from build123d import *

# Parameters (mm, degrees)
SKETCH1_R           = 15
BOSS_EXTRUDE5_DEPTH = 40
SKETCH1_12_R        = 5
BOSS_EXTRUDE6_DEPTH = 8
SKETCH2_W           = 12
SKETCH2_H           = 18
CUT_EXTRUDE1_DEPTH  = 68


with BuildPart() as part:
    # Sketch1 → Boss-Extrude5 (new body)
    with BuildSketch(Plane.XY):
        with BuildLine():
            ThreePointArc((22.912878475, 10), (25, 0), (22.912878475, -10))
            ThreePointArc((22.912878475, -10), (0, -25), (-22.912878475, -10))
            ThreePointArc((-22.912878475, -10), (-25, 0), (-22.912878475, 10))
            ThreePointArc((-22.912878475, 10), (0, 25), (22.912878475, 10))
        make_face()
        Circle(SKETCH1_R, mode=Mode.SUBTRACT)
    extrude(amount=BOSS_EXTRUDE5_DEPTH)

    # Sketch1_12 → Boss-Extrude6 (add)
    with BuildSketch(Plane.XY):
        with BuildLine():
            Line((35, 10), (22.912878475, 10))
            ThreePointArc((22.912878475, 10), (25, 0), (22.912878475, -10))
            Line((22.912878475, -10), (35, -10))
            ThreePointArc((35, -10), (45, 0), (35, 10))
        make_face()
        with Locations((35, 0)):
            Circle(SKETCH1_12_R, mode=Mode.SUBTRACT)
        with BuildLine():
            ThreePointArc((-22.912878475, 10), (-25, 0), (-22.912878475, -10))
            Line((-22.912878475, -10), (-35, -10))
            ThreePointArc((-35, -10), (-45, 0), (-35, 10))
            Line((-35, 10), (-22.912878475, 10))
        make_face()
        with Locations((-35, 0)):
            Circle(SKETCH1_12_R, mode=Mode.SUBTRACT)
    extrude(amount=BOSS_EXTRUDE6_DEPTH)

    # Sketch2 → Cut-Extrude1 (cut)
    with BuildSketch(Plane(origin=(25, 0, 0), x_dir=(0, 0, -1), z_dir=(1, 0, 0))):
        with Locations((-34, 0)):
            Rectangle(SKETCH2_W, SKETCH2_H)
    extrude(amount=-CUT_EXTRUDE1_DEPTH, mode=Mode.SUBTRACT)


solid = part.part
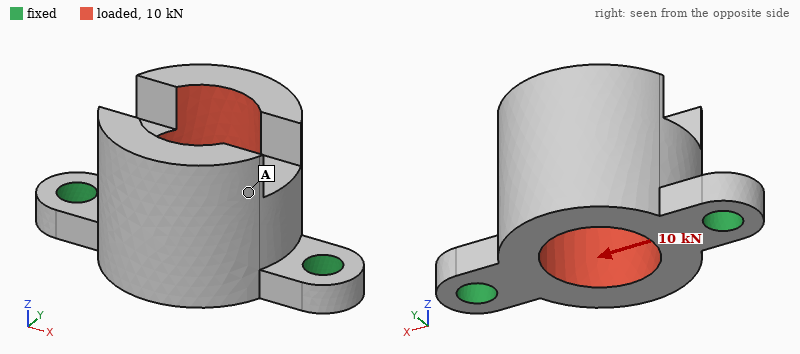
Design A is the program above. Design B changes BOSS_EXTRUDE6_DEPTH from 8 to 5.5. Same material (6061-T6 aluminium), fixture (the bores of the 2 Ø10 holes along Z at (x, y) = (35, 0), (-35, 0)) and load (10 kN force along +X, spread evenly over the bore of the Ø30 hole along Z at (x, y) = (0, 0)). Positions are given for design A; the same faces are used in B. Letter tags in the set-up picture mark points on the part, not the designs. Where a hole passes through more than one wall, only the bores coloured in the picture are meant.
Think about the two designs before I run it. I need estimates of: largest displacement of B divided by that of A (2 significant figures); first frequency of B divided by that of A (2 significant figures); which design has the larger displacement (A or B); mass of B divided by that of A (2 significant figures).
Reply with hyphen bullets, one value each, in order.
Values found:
- 1.5
- 0.68
- B
- 0.97
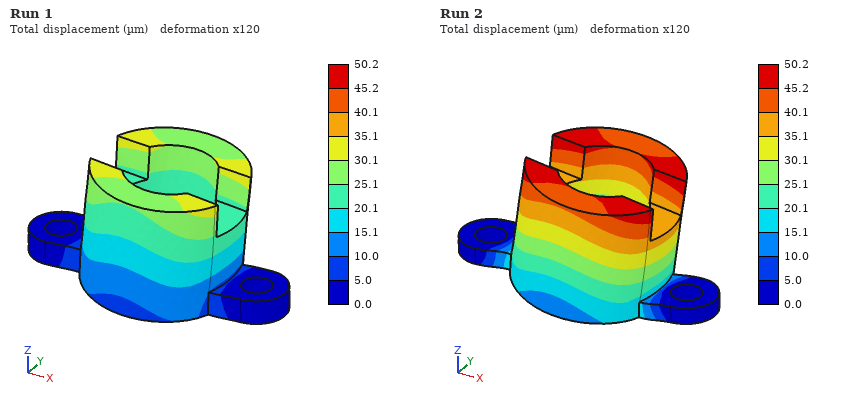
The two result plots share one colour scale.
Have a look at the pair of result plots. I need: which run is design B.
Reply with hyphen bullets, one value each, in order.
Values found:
- Run 2
